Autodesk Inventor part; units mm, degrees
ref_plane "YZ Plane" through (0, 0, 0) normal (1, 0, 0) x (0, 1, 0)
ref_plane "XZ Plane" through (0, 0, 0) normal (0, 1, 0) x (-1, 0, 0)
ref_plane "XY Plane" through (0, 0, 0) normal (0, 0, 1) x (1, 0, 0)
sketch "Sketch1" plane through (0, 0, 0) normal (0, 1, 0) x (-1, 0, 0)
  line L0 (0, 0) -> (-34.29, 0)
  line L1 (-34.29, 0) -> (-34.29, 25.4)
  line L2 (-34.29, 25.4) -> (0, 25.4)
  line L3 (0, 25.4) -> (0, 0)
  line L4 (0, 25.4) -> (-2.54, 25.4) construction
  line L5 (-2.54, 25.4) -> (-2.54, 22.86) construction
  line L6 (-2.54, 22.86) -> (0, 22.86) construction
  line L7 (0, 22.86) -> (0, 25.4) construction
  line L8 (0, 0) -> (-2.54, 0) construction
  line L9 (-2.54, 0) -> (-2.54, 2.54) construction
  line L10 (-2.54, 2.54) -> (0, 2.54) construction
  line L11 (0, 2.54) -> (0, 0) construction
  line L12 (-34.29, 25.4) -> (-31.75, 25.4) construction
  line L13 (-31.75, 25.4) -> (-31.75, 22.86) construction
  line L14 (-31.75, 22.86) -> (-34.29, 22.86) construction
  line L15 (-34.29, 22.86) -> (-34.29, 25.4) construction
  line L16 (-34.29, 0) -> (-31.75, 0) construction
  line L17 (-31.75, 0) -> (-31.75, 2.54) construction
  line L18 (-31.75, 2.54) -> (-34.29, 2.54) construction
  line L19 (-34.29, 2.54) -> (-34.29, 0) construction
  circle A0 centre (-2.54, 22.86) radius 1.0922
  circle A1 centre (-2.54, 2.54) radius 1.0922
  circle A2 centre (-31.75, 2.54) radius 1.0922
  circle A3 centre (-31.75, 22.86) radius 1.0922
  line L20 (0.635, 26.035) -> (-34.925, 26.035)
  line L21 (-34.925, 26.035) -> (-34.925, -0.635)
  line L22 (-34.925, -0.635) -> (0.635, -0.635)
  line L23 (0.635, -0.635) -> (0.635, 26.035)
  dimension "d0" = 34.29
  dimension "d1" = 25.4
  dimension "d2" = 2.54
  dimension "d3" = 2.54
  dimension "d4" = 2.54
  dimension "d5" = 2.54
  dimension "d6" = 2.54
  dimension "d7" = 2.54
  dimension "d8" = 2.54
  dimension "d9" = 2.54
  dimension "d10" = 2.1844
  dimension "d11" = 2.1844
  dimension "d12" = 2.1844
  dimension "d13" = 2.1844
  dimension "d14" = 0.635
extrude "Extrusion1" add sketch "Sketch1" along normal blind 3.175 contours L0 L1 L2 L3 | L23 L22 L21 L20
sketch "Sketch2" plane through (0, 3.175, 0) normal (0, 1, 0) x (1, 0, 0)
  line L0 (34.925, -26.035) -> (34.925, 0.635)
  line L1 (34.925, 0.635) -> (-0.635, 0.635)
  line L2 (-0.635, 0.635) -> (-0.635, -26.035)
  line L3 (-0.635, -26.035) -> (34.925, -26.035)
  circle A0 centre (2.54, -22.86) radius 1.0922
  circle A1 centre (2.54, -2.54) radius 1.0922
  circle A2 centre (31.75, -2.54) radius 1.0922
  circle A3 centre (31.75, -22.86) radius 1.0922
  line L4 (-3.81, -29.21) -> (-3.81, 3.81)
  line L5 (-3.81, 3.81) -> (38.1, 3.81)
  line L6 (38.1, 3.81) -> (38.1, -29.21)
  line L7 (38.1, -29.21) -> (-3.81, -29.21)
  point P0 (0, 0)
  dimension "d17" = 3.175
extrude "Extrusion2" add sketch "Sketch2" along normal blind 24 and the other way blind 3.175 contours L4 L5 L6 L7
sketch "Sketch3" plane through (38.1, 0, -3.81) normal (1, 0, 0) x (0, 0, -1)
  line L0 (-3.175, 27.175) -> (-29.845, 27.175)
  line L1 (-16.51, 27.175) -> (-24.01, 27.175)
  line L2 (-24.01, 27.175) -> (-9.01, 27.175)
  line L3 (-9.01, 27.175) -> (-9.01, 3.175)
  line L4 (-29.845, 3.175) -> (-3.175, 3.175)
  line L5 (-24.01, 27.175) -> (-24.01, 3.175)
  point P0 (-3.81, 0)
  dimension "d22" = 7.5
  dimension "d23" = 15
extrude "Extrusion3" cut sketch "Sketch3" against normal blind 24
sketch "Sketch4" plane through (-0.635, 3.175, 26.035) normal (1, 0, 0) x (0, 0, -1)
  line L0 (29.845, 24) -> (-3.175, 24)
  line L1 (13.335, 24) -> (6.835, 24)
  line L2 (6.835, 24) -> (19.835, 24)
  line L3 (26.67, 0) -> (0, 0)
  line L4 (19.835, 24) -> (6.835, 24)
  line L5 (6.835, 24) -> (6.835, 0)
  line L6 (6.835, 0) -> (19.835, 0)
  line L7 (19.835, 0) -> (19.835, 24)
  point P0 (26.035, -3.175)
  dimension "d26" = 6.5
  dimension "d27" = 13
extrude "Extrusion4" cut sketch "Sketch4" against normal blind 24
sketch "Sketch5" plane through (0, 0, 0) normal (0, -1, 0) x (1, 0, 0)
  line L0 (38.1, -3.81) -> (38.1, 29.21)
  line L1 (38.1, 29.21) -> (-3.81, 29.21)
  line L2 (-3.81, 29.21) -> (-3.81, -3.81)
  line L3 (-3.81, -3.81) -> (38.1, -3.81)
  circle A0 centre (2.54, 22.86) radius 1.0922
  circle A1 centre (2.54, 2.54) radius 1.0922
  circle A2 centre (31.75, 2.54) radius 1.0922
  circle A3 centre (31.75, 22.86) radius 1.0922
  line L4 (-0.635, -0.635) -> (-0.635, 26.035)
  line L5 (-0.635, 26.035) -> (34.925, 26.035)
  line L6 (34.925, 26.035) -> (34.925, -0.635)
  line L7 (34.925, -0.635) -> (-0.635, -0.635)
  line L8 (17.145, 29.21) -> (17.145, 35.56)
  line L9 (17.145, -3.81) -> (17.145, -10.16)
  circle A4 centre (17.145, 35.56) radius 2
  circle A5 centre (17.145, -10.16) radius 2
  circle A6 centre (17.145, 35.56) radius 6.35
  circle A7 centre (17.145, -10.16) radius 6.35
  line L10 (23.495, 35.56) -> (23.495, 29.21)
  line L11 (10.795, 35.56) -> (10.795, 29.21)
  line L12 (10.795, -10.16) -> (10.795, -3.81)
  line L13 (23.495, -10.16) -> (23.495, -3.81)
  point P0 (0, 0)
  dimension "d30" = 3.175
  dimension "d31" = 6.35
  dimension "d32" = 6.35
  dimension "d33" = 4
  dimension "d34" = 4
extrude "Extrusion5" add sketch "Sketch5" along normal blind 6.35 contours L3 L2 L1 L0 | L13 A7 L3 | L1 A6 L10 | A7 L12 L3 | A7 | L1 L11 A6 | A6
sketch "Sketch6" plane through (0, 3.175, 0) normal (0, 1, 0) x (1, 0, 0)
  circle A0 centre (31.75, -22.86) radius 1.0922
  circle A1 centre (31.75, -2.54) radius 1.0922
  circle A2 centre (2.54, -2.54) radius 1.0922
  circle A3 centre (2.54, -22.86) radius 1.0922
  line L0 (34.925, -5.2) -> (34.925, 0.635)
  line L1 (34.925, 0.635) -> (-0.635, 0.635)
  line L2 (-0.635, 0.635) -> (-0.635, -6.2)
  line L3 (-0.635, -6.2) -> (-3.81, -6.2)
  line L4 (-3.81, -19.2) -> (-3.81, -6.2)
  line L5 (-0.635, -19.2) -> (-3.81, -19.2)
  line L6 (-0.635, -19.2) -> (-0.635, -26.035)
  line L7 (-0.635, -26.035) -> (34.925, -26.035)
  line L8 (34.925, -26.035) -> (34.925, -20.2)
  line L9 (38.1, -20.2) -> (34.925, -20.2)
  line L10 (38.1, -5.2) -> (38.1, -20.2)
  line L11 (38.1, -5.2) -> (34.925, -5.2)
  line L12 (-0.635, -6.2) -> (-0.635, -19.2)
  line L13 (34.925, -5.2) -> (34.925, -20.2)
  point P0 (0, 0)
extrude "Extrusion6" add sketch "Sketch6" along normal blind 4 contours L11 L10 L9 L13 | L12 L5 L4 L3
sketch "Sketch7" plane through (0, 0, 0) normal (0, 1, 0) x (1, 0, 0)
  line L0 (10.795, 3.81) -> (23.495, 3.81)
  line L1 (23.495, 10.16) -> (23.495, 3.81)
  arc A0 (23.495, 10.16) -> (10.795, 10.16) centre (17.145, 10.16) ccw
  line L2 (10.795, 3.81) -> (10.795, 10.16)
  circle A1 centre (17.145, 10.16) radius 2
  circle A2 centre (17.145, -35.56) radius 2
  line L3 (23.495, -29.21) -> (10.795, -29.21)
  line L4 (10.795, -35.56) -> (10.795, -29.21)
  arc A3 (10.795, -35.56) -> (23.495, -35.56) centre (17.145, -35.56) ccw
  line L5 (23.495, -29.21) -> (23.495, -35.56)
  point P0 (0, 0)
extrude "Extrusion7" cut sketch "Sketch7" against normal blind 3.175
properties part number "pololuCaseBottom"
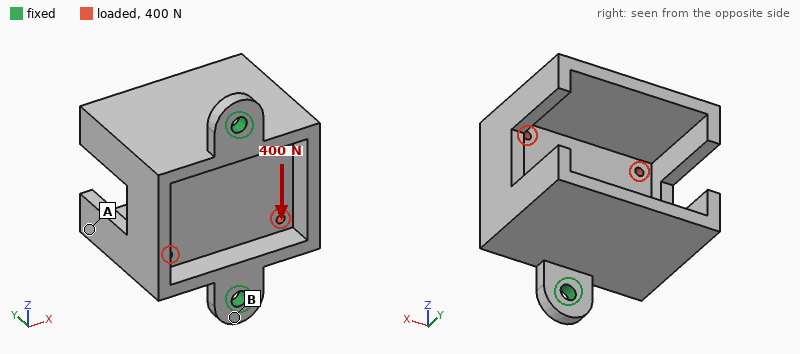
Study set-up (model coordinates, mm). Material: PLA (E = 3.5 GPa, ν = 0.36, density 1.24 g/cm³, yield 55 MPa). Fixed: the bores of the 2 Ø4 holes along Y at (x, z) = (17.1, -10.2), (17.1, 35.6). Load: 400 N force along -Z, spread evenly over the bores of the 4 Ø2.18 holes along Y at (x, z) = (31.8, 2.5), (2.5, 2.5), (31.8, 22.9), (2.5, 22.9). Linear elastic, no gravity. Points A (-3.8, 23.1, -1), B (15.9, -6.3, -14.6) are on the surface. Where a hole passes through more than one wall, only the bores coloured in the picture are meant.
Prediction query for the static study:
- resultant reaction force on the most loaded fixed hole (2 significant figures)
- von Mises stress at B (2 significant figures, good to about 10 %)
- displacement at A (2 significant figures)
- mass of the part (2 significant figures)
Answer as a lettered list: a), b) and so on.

a) 210 N
b) 2.4 MPa
c) 74 µm
d) 21 g
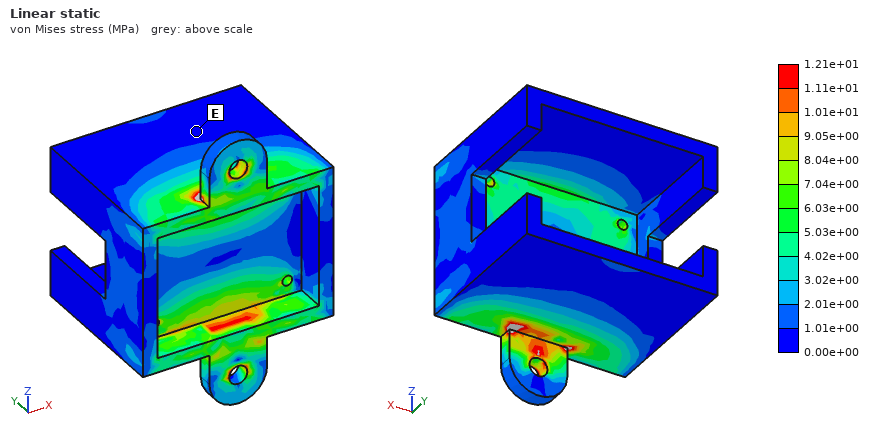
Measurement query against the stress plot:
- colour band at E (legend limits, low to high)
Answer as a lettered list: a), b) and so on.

a) 0.00e+00 to 1.01e+00 MPa
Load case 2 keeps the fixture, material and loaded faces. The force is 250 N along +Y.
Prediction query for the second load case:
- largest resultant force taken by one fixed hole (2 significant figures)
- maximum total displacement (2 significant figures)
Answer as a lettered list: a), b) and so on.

a) 150 N
b) 87 µm
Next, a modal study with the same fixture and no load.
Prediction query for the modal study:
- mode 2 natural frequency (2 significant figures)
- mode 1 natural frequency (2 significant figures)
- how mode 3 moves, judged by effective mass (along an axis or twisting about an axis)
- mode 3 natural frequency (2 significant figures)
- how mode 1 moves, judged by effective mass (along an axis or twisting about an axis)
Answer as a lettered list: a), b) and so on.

a) 1300 Hz
b) 440 Hz
c) along Z
d) 1700 Hz
e) along X
